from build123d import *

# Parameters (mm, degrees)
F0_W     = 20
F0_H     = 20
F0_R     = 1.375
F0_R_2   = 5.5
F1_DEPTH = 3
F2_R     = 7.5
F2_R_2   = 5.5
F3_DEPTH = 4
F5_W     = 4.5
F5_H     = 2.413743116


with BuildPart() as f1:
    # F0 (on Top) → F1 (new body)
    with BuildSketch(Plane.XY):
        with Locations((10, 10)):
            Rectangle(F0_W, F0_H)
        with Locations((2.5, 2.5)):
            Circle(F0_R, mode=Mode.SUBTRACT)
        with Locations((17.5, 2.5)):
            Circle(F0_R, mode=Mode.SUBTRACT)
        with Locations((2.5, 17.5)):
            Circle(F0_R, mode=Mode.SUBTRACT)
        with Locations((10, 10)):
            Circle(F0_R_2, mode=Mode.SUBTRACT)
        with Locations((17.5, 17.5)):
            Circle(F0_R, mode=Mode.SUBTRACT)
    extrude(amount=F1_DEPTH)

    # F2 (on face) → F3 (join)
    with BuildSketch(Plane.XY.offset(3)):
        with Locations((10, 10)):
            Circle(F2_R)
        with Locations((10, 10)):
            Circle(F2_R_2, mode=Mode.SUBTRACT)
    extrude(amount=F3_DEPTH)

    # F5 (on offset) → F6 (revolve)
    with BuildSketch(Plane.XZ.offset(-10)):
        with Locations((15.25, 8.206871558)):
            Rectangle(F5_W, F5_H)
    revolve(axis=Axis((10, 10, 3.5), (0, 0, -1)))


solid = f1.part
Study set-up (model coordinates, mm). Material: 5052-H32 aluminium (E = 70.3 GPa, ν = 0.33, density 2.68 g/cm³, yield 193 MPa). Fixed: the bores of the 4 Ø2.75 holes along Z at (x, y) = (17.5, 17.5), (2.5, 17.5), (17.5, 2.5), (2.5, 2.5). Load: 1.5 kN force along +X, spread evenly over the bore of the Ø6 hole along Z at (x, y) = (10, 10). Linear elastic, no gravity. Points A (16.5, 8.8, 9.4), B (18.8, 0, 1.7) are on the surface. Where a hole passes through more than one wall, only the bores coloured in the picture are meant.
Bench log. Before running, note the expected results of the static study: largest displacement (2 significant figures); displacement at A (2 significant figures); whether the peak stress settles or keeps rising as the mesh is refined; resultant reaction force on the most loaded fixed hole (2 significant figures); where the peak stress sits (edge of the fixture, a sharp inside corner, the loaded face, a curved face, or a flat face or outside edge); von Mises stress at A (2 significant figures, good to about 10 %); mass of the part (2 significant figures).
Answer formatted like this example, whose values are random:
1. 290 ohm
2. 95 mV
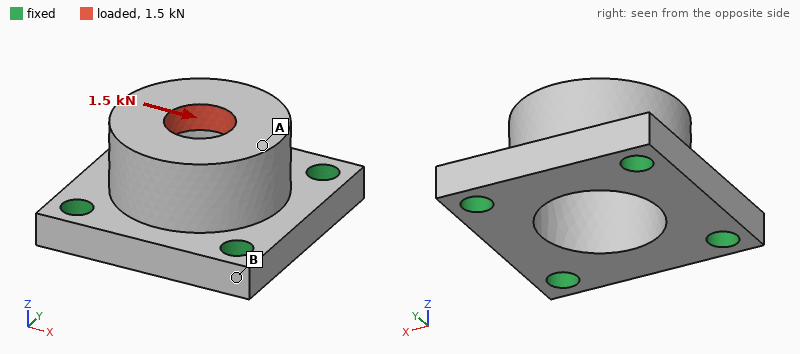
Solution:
1. 18 µm
2. 17 µm
3. keeps rising
4. 530 N
5. edge of the fixture
6. 43 MPa
7. 4.1 g
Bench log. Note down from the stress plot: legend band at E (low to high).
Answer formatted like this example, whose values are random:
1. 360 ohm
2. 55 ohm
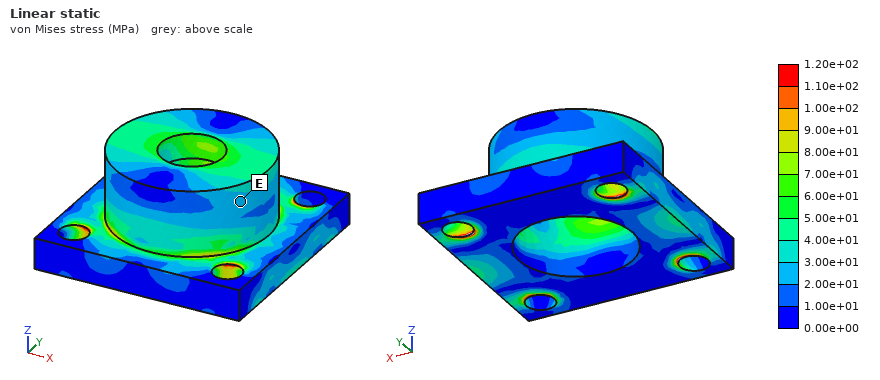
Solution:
1. 2.00e+01 to 3.00e+01 MPa
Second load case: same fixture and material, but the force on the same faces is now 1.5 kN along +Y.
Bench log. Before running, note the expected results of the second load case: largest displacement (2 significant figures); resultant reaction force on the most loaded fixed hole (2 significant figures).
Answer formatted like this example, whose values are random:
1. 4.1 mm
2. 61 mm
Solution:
1. 18 µm
2. 530 N
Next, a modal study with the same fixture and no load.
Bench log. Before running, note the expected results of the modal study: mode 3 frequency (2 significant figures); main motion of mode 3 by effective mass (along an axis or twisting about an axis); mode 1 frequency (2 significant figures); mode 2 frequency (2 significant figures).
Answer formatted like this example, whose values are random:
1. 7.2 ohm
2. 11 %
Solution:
1. 51 kHz
2. along Z
3. 44 kHz
4. 44 kHz
